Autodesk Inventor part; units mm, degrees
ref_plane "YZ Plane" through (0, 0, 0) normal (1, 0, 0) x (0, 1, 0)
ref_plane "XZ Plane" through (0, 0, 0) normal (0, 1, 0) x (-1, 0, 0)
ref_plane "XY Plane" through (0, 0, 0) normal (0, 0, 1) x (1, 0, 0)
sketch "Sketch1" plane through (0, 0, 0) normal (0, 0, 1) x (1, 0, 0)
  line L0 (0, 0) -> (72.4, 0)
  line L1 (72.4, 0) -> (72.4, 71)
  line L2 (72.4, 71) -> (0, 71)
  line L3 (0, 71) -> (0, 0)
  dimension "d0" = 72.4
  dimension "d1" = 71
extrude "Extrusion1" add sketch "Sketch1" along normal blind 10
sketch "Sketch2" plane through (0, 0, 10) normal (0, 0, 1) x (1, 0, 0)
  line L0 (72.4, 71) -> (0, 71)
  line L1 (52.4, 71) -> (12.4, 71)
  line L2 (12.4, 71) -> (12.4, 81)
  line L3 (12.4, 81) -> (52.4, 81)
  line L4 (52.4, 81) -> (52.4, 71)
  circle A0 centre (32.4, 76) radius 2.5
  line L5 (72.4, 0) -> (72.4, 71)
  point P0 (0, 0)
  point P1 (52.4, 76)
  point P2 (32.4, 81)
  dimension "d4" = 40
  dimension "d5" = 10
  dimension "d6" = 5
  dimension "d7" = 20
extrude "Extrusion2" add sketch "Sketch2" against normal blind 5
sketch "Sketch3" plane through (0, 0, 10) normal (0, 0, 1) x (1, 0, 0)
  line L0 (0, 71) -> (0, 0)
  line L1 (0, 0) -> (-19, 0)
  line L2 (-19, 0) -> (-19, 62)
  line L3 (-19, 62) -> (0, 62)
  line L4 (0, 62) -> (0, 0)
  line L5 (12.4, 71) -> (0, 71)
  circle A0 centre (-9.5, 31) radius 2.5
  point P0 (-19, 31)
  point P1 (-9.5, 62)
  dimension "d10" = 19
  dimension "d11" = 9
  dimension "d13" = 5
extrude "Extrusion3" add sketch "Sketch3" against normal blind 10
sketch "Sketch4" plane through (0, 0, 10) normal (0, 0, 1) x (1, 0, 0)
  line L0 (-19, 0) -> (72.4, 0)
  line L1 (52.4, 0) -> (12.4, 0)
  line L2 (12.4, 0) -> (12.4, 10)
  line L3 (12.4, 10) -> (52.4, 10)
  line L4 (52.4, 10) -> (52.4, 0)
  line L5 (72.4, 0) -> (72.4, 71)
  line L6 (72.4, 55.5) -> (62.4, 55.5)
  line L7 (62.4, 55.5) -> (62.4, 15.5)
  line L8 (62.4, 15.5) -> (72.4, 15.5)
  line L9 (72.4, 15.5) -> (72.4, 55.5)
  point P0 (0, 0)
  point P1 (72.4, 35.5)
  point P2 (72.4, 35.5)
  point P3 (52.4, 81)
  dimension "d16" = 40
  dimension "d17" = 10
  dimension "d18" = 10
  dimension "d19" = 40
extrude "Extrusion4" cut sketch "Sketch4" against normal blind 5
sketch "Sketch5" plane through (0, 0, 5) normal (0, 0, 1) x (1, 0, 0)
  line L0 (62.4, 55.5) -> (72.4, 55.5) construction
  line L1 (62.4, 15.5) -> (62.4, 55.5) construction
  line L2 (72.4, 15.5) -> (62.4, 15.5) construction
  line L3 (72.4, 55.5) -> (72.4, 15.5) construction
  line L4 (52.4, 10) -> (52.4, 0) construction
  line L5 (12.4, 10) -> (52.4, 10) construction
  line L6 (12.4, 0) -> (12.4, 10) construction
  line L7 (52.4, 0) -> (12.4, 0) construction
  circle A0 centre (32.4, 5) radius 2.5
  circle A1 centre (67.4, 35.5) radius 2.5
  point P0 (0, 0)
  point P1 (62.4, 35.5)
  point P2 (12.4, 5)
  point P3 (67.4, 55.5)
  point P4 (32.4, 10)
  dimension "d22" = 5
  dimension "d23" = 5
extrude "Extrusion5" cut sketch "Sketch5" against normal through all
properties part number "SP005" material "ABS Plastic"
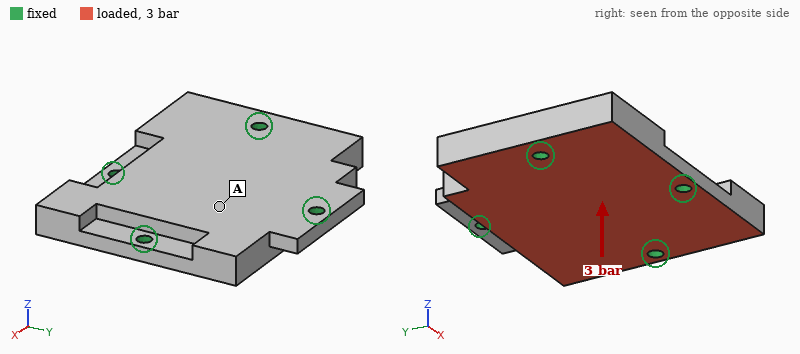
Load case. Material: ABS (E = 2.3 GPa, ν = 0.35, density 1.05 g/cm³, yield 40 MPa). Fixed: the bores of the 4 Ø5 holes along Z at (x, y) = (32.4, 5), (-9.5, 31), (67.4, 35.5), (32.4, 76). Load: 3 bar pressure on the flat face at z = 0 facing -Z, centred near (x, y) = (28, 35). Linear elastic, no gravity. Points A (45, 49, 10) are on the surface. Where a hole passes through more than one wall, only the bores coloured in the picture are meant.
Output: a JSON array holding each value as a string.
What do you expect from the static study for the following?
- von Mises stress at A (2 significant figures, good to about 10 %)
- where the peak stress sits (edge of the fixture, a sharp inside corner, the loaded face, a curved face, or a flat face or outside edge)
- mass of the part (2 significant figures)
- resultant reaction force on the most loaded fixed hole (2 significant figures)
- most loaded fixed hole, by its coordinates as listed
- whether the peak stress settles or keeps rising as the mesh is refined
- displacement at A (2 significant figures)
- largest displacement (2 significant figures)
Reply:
["3.0 MPa", "edge of the fixture", "64 g", "640 N", "(-9.5, 31)", "keeps rising", "0.14 mm", "0.24 mm"]
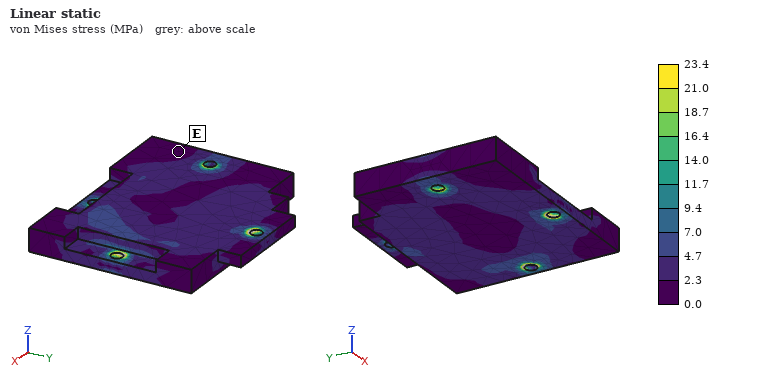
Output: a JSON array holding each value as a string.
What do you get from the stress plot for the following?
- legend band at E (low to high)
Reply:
["0.0 to 2.3 MPa"]
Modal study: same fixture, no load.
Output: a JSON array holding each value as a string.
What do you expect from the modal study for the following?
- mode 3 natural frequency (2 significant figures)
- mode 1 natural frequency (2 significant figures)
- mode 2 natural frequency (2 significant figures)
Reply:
["2300 Hz", "2000 Hz", "2200 Hz"]
